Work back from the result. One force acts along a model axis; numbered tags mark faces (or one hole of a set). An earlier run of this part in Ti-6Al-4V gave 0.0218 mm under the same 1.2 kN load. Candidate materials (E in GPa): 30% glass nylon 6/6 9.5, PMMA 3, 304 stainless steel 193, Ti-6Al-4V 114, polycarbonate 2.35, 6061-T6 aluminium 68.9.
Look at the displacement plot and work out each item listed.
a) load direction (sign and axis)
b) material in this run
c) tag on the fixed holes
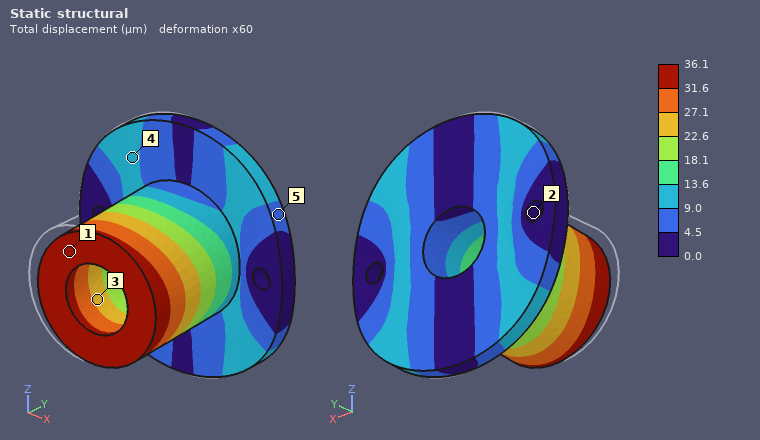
+X
6061-T6 aluminium
2
